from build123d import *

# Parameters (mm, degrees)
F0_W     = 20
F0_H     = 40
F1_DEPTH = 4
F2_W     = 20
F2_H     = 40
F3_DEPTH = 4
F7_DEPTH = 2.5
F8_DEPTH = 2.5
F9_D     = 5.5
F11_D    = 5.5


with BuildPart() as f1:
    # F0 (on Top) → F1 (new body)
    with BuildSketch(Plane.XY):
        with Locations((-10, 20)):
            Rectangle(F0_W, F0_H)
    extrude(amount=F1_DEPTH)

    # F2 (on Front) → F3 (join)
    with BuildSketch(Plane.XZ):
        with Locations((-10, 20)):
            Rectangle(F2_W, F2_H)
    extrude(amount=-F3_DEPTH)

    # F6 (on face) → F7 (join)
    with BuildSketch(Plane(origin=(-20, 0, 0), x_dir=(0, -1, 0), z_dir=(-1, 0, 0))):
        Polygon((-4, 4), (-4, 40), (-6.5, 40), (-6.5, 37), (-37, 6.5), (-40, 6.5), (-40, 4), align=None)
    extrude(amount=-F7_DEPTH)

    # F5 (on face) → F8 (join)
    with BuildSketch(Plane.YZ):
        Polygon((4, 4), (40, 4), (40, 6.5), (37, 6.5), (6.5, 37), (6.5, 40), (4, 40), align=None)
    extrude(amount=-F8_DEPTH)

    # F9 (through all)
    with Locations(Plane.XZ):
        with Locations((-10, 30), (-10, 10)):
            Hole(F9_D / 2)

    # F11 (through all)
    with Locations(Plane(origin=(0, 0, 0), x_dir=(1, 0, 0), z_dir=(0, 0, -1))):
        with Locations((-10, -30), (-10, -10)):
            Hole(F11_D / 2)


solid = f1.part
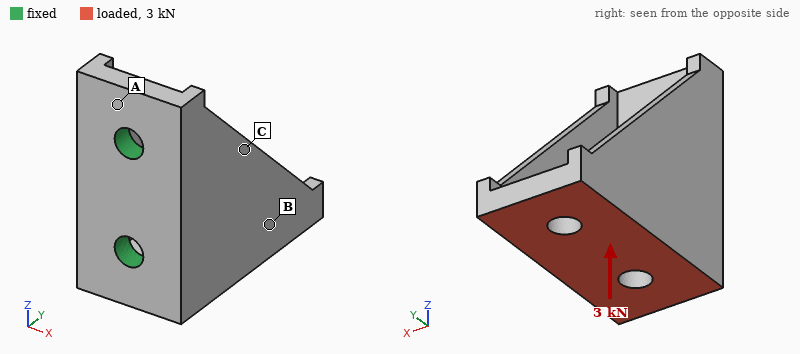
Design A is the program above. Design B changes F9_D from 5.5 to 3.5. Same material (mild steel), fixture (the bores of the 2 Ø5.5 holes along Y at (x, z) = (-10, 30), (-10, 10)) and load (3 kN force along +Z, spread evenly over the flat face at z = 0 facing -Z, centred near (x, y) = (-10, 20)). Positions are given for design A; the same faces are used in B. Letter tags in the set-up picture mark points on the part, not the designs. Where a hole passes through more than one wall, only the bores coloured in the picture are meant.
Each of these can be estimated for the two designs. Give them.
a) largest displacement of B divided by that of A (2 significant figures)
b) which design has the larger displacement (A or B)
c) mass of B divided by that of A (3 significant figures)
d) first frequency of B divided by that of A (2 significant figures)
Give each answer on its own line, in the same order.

1.2
B
1.01
0.84
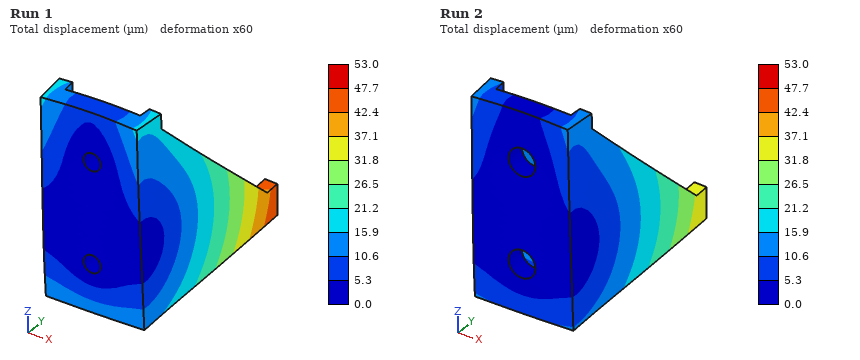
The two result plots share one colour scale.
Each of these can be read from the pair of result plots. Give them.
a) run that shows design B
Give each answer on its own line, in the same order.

Run 1
